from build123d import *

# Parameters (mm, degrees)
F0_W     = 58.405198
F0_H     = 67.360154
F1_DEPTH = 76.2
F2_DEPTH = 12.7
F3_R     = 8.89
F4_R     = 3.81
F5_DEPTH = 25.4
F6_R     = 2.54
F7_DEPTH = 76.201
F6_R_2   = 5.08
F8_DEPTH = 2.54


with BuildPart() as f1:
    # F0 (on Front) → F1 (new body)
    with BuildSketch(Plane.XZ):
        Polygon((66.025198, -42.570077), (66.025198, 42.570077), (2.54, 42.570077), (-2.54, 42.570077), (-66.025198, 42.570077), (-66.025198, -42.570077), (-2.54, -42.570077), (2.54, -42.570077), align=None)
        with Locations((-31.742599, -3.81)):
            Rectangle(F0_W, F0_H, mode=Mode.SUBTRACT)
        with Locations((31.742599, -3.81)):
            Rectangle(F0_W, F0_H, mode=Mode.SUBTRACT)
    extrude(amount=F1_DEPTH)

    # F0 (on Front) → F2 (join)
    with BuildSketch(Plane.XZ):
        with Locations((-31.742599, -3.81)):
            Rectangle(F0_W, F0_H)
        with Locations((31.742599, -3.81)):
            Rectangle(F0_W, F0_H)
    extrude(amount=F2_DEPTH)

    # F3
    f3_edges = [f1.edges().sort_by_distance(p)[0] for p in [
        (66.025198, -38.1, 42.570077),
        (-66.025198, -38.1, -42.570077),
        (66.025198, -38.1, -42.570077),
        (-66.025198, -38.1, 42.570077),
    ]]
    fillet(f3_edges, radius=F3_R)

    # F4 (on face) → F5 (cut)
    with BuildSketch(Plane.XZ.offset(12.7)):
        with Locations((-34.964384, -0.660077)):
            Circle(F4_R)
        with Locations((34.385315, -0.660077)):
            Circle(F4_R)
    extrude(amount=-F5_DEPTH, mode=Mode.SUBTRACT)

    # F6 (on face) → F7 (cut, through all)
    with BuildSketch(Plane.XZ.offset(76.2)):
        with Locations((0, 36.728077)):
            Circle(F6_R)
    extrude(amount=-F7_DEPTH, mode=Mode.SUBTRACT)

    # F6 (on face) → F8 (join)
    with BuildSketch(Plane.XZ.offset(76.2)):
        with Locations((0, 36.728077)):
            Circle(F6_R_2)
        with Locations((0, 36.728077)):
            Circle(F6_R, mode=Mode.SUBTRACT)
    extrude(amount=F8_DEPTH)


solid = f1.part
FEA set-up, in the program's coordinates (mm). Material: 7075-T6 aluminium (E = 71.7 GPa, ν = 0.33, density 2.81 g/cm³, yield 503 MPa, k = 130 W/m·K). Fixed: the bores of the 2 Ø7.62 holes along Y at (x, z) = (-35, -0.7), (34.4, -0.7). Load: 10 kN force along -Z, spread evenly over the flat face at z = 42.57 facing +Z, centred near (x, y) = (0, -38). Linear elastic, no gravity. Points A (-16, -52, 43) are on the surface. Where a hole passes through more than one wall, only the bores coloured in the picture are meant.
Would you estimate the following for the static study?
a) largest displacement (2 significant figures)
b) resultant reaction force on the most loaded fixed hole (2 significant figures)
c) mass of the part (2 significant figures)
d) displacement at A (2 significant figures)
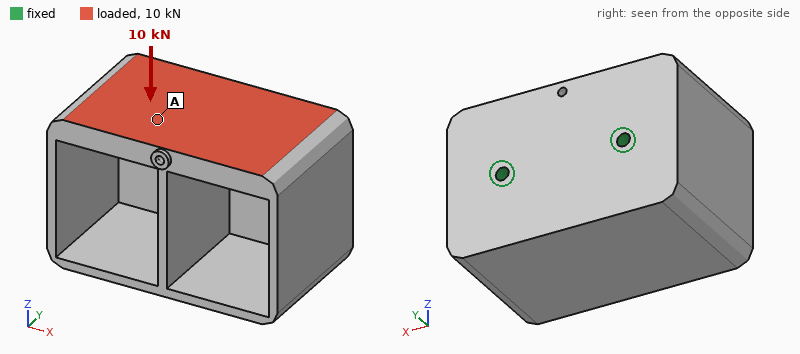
0.25 mm
5.1 kN
980 g
0.19 mm
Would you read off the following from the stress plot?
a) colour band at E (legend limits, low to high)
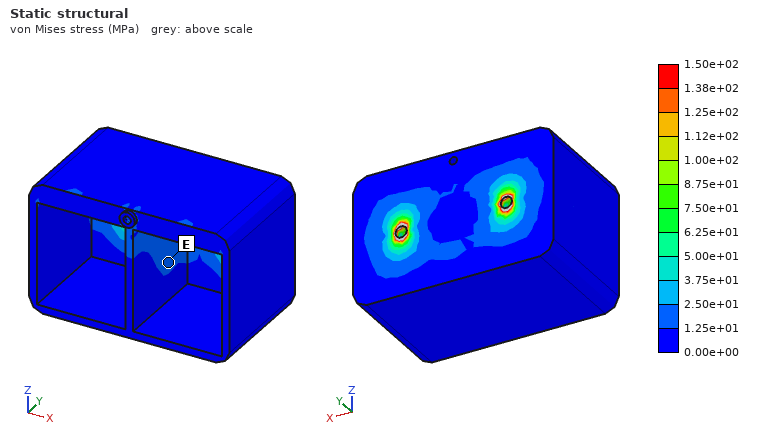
1.25e+01 to 2.50e+01 MPa
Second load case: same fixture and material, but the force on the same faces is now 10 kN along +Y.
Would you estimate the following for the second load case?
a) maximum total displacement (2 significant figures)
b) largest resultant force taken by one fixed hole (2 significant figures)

0.32 mm
5.0 kN
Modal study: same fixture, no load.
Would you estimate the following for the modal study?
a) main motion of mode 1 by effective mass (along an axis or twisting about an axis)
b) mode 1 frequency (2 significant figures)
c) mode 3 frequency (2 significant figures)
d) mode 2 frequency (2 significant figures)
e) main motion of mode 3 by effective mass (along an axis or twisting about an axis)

along Z
1200 Hz
2600 Hz
1900 Hz
along X
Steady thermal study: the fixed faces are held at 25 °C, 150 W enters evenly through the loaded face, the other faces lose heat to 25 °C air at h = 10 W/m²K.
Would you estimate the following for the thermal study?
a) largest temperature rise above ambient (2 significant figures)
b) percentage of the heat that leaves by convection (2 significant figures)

37 K
9.3 %
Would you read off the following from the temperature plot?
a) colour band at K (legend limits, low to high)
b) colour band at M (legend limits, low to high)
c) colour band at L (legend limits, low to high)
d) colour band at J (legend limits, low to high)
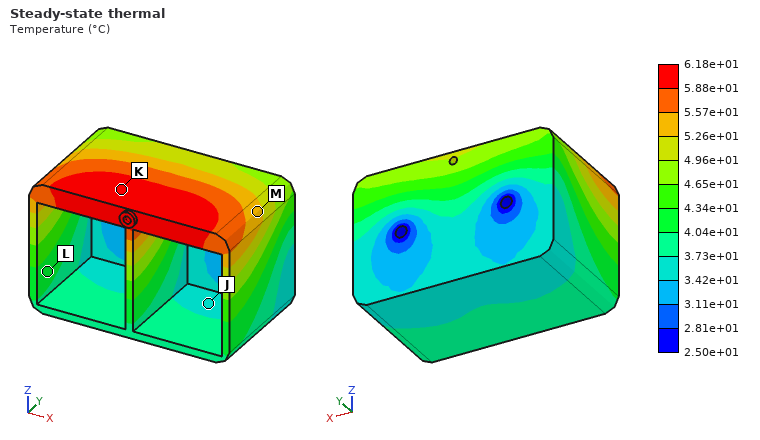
5.88e+01 to 6.18e+01 °C
5.26e+01 to 5.57e+01 °C
4.04e+01 to 4.34e+01 °C
3.42e+01 to 3.73e+01 °C
